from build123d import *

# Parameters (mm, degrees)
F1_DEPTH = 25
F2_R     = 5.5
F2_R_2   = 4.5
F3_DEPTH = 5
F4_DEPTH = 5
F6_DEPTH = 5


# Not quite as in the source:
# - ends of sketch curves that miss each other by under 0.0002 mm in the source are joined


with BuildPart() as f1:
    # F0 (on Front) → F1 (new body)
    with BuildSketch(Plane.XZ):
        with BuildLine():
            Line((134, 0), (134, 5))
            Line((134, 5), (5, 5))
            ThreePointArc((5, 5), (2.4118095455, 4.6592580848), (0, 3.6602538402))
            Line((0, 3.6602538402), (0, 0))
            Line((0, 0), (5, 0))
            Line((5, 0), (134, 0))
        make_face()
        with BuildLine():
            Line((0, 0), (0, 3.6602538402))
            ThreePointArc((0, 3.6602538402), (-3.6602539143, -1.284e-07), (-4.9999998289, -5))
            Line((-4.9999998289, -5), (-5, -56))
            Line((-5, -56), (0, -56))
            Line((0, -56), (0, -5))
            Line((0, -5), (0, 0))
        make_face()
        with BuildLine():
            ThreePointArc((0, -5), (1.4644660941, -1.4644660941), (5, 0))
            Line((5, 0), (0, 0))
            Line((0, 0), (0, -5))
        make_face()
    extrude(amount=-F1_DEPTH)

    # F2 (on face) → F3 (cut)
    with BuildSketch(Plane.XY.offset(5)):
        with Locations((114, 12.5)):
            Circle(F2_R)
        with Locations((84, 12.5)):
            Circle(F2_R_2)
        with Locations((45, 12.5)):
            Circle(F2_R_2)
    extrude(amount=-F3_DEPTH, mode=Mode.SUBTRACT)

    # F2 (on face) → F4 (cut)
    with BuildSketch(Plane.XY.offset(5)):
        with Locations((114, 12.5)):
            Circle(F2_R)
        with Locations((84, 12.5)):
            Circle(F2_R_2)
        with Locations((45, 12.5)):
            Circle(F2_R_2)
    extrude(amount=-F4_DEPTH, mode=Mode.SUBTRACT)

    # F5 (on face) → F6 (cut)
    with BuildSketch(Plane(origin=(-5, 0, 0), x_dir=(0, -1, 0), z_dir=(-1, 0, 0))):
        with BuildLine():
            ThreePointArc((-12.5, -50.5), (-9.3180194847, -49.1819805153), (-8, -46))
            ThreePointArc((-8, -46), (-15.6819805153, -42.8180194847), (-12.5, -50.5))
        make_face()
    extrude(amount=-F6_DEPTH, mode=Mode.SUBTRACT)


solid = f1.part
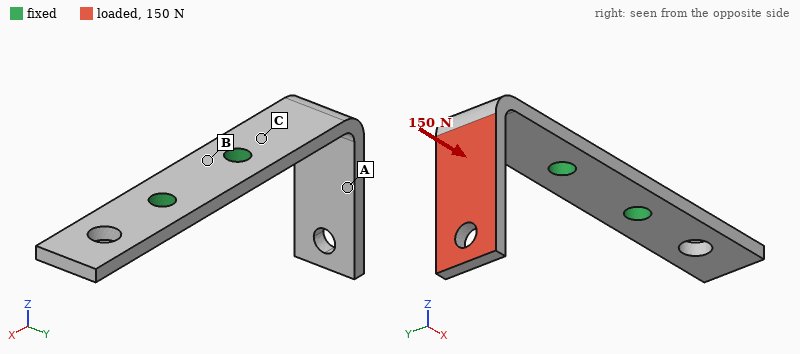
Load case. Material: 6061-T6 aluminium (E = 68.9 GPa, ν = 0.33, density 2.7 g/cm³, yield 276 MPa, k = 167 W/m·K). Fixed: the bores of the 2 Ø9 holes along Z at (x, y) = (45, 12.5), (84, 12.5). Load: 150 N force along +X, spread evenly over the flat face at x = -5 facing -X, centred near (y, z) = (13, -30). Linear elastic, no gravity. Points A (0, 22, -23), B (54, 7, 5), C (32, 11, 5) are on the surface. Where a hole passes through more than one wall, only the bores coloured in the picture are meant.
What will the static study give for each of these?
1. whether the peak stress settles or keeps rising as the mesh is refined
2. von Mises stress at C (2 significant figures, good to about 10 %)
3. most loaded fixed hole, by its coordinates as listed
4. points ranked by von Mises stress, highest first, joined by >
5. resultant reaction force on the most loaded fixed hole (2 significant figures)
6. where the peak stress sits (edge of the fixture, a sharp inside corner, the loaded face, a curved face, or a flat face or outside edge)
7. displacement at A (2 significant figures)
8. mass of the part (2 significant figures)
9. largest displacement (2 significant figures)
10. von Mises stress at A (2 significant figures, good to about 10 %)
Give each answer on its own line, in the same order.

keeps rising
42 MPa
(45, 12.5)
C > A > B
140 N
edge of the fixture
0.41 mm
61 g
0.91 mm
15 MPa
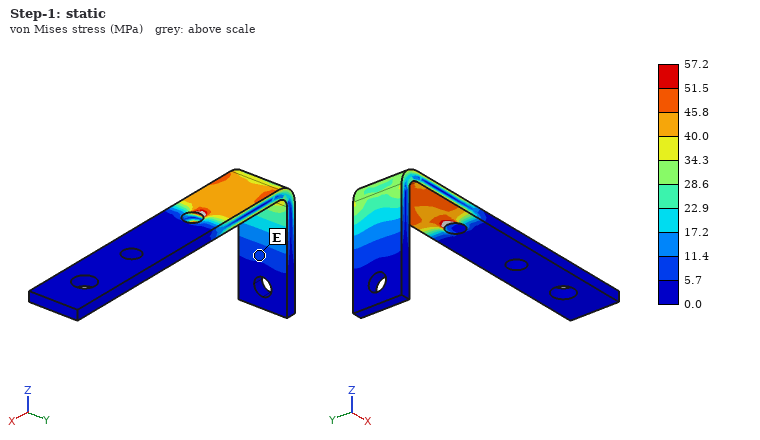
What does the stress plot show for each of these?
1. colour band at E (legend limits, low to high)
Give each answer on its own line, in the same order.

5.7 to 11.4 MPa
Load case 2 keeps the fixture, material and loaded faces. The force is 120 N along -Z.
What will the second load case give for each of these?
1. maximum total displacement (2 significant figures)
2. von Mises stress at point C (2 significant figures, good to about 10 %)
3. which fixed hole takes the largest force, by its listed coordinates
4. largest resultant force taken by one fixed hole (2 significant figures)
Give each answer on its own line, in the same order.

0.50 mm
39 MPa
(45, 12.5)
120 N
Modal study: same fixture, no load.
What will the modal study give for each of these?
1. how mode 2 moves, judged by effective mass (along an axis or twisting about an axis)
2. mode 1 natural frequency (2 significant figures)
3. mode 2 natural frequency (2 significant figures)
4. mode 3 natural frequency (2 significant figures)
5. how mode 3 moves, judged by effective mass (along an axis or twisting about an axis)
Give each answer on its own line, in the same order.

along Y
540 Hz
820 Hz
1600 Hz
along Z
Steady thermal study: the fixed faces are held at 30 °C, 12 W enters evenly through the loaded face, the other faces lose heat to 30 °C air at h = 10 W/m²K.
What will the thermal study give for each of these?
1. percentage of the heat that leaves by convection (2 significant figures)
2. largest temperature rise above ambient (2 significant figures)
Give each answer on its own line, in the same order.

9.3 %
40 K
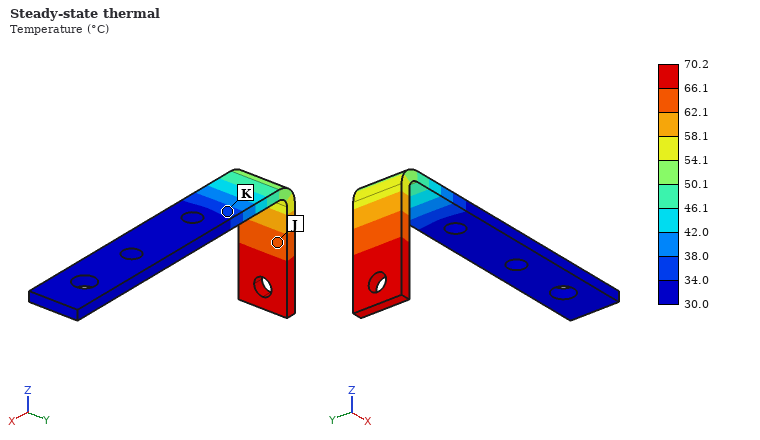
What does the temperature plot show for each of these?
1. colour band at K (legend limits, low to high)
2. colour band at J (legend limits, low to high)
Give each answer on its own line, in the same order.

34.0 to 38.0 °C
62.1 to 66.1 °C
